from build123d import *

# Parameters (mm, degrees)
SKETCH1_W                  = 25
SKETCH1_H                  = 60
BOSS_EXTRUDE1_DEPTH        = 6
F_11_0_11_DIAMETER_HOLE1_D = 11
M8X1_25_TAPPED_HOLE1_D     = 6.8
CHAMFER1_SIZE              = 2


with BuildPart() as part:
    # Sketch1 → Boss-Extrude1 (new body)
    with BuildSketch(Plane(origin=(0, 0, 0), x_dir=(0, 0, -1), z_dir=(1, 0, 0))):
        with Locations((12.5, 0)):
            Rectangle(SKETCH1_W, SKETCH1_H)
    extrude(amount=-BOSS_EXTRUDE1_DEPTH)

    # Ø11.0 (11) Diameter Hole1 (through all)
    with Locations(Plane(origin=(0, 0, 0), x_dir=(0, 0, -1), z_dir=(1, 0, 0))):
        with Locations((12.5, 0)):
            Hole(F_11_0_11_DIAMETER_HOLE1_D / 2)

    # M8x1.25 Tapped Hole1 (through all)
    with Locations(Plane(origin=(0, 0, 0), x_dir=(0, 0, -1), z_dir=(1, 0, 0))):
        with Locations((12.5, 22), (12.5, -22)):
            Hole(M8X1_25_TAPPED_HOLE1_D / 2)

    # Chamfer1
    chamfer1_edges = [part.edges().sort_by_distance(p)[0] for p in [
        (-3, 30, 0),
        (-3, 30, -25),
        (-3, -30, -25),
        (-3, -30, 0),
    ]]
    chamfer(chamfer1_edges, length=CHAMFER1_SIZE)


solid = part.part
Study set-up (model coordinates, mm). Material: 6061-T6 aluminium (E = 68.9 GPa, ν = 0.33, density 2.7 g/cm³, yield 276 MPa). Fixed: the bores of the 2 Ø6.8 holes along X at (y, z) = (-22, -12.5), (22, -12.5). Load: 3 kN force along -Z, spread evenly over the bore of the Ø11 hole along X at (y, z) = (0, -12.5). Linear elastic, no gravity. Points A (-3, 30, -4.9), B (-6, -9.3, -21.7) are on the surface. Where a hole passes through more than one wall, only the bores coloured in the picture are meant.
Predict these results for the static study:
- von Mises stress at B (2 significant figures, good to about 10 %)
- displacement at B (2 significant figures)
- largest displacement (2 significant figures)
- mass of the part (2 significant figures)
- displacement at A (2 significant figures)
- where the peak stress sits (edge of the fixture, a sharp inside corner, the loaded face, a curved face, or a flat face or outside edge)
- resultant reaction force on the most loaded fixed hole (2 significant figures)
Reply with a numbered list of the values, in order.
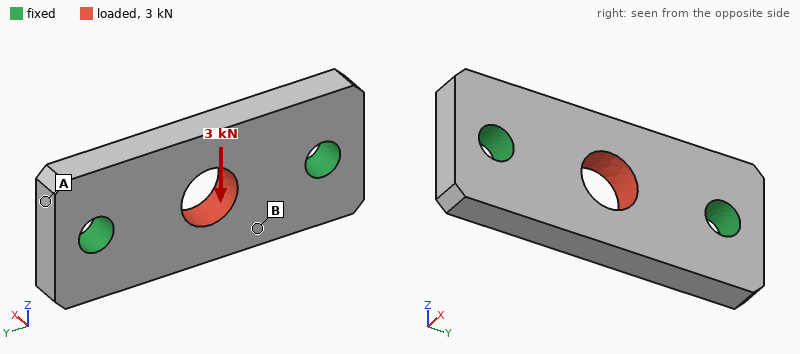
1. 18 MPa
2. 8.8 µm
3. 14 µm
4. 21 g
5. 2.9 µm
6. edge of the fixture
7. 1.5 kN
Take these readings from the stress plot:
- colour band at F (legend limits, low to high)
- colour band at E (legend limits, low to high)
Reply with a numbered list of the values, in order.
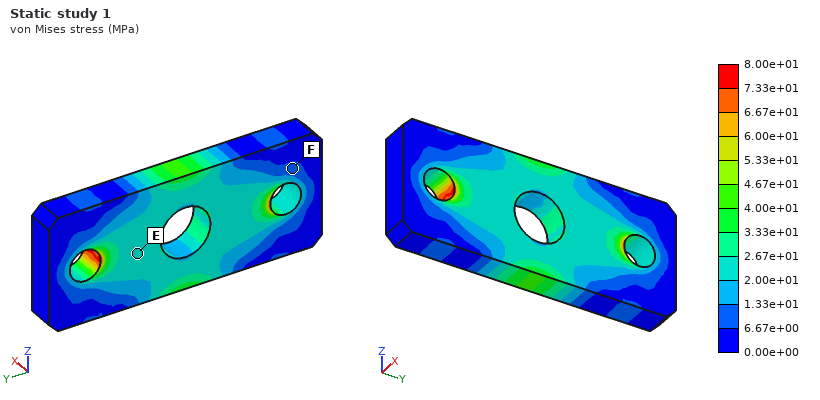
1. 6.67e+00 to 1.33e+01 MPa
2. 2.00e+01 to 2.67e+01 MPa
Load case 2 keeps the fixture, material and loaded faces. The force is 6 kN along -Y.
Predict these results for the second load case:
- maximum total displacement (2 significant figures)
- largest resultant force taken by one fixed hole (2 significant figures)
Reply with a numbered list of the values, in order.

1. 8.5 µm
2. 3.0 kN
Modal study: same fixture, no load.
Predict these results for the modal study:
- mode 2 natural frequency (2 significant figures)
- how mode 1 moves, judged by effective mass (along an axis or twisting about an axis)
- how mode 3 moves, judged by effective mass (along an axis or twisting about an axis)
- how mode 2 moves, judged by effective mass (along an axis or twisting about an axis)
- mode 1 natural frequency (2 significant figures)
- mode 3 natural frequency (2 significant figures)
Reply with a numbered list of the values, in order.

1. 17 kHz
2. along X
3. along Z
4. twisting about Y
5. 16 kHz
6. 28 kHz
